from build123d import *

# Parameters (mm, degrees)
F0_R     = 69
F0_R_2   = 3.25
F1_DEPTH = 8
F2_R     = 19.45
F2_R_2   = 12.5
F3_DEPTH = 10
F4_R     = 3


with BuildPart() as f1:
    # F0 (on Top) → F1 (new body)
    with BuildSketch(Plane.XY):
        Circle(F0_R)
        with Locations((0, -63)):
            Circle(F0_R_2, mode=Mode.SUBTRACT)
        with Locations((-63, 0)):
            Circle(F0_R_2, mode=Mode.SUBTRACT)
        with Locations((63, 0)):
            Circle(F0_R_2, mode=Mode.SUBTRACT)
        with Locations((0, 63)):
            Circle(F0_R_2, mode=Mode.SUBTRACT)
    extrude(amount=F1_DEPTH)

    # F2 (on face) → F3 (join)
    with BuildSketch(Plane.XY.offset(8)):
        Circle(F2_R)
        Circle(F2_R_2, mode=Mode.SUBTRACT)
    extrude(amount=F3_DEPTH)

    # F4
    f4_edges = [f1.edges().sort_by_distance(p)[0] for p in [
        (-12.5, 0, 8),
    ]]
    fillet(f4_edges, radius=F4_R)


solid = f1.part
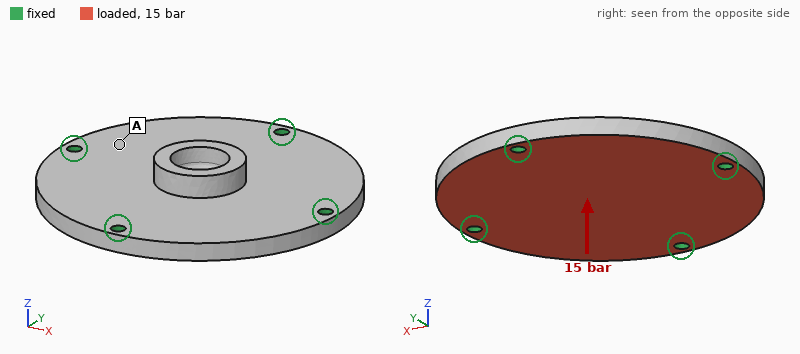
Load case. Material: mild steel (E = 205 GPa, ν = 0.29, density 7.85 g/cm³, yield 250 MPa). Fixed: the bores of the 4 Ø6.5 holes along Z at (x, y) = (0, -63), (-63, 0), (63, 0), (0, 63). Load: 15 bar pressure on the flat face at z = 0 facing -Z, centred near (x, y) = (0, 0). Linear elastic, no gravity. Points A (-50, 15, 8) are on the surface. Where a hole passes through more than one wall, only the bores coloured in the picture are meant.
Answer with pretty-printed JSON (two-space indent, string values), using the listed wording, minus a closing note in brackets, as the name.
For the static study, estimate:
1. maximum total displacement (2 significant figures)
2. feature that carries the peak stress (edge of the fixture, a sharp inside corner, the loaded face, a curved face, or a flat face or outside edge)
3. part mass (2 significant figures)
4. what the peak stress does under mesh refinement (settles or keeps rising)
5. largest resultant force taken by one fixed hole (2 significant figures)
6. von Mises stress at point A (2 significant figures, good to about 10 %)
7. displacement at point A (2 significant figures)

{
  "maximum total displacement": "62 µm",
  "feature that carries the peak stress": "edge of the fixture",
  "part mass": "990 g",
  "what the peak stress does under mesh refinement": "keeps rising",
  "largest resultant force taken by one fixed hole": "5.6 kN",
  "von Mises stress at point A": "35 MPa",
  "displacement at point A": "24 µm"
}
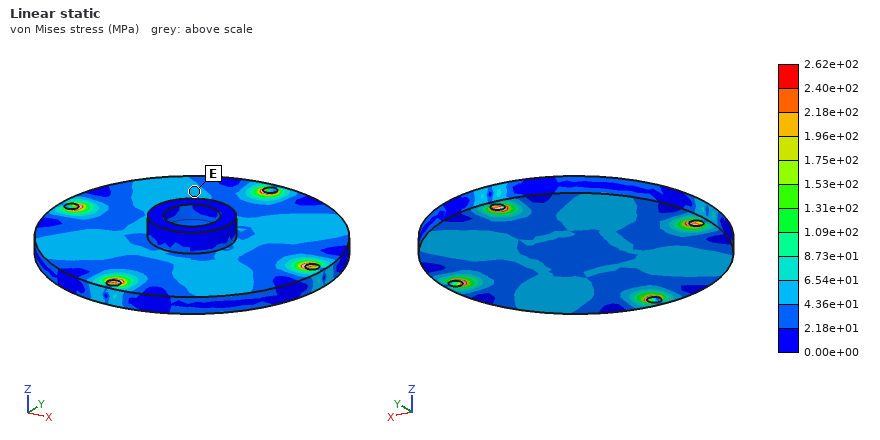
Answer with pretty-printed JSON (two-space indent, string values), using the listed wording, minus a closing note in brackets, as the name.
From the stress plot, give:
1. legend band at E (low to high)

{
  "legend band at E": "4.36e+01 to 6.54e+01 MPa"
}
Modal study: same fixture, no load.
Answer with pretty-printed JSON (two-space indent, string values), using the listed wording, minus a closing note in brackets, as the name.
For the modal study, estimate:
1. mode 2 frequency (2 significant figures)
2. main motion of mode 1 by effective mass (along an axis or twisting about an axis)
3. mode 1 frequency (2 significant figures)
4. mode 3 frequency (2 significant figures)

{
  "mode 2 frequency": "4400 Hz",
  "main motion of mode 1 by effective mass": "along Z",
  "mode 1 frequency": "3400 Hz",
  "mode 3 frequency": "4500 Hz"
}
